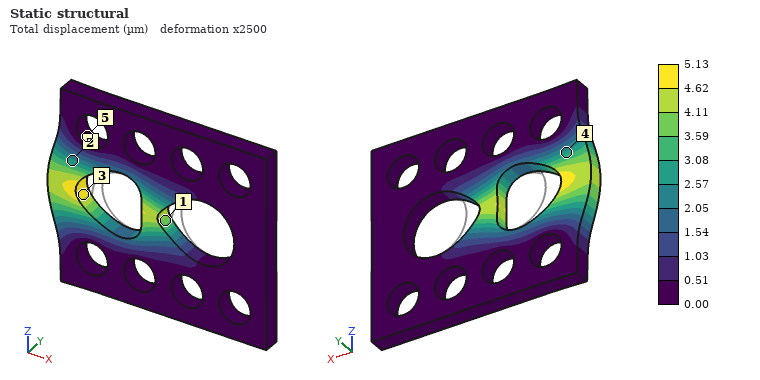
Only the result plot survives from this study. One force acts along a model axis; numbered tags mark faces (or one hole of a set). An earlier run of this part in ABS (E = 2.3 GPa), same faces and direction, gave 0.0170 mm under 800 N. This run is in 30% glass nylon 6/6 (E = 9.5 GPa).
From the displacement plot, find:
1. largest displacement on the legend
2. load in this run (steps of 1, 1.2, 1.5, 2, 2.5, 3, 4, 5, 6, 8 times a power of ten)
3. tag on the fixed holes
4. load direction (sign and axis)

5.13 µm
1 kN
5
-X
